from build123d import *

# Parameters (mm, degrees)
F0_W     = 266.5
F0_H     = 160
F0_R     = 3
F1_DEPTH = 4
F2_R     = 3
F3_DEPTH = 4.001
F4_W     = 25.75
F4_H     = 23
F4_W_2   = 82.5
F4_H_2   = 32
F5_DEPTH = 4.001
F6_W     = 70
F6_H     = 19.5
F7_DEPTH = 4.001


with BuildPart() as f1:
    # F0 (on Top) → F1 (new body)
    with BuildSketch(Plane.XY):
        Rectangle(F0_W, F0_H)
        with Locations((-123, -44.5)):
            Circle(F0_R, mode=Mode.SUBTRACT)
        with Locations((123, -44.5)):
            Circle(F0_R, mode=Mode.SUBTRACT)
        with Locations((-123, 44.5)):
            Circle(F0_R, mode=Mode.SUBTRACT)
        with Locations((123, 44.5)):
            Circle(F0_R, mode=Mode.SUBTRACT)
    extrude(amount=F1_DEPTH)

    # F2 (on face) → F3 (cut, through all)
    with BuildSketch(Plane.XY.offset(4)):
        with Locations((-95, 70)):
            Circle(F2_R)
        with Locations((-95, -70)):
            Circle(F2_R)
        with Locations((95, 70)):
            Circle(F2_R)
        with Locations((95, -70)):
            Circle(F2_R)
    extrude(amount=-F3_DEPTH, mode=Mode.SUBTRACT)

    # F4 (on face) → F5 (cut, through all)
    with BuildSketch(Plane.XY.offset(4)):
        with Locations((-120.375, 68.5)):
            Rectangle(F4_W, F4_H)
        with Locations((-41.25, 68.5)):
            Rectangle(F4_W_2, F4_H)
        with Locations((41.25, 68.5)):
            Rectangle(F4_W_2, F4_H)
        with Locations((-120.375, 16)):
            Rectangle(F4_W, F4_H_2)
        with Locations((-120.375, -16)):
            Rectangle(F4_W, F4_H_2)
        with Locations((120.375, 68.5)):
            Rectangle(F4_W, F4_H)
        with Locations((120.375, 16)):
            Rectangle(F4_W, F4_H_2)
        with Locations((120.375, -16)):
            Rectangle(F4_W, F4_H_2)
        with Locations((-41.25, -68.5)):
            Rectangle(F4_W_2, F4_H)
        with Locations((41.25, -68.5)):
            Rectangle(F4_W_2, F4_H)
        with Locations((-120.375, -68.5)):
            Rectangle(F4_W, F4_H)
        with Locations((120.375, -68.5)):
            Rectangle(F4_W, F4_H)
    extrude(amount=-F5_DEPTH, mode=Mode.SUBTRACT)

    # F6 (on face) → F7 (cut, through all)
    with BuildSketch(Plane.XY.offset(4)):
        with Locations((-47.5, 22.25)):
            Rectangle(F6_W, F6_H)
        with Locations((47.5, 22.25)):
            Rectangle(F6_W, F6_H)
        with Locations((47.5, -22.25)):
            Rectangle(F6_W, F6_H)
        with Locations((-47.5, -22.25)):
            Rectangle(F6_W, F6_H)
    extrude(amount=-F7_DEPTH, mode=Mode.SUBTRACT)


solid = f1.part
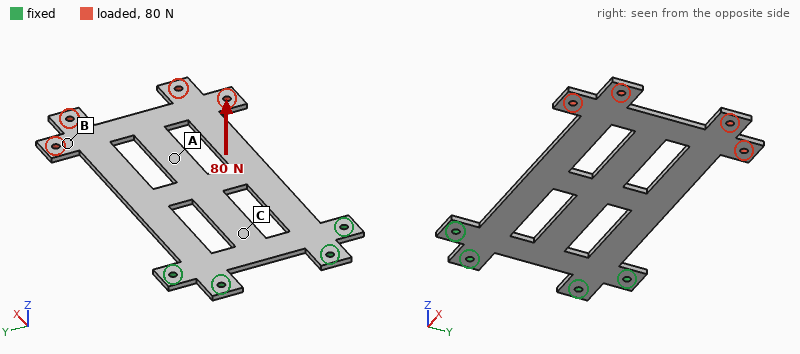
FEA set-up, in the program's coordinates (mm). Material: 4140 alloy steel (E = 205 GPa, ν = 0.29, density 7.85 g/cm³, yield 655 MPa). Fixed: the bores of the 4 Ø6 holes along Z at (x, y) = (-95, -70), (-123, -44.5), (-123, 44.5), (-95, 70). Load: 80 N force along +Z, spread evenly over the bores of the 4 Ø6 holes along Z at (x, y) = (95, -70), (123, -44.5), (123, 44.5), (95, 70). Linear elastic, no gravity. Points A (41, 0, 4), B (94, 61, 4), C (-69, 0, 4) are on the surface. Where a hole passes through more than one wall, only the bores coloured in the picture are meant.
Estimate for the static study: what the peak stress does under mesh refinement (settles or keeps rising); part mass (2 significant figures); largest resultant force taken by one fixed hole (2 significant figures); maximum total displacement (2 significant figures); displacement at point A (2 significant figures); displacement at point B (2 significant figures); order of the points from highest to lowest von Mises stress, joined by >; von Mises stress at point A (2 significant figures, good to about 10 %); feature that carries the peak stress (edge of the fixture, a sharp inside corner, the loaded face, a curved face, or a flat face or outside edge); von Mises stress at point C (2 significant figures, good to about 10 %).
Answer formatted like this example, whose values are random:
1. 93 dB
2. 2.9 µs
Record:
1. keeps rising
2. 740 g
3. 190 N
4. 3.6 mm
5. 1.7 mm
6. 2.7 mm
7. C > A > B
8. 28 MPa
9. edge of the fixture
10. 60 MPa
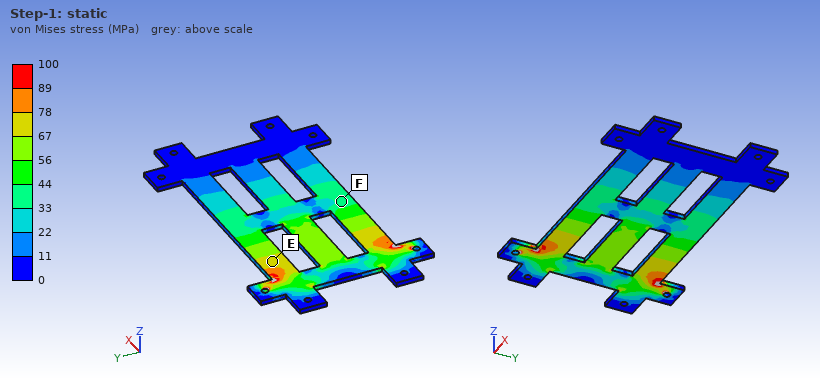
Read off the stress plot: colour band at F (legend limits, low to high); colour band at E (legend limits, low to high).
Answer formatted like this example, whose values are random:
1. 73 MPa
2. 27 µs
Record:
1. 33 to 44 MPa
2. 67 to 78 MPa
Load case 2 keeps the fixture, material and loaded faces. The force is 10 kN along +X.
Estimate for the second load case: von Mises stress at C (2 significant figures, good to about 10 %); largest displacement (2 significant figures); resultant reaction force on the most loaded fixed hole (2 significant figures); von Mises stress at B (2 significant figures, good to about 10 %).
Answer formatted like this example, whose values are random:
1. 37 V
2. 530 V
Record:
1. 19 MPa
2. 91 µm
3. 4.1 kN
4. 65 MPa
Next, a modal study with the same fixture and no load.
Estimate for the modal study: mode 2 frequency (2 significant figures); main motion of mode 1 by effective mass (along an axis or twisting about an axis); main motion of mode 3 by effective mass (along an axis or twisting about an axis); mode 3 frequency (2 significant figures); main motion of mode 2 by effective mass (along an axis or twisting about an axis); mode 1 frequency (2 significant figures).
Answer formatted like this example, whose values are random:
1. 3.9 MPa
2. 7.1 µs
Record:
1. 200 Hz
2. along Z
3. along Z
4. 360 Hz
5. twisting about X
6. 55 Hz
